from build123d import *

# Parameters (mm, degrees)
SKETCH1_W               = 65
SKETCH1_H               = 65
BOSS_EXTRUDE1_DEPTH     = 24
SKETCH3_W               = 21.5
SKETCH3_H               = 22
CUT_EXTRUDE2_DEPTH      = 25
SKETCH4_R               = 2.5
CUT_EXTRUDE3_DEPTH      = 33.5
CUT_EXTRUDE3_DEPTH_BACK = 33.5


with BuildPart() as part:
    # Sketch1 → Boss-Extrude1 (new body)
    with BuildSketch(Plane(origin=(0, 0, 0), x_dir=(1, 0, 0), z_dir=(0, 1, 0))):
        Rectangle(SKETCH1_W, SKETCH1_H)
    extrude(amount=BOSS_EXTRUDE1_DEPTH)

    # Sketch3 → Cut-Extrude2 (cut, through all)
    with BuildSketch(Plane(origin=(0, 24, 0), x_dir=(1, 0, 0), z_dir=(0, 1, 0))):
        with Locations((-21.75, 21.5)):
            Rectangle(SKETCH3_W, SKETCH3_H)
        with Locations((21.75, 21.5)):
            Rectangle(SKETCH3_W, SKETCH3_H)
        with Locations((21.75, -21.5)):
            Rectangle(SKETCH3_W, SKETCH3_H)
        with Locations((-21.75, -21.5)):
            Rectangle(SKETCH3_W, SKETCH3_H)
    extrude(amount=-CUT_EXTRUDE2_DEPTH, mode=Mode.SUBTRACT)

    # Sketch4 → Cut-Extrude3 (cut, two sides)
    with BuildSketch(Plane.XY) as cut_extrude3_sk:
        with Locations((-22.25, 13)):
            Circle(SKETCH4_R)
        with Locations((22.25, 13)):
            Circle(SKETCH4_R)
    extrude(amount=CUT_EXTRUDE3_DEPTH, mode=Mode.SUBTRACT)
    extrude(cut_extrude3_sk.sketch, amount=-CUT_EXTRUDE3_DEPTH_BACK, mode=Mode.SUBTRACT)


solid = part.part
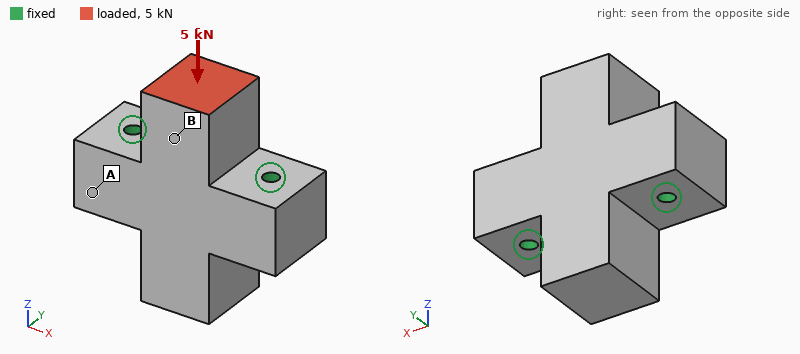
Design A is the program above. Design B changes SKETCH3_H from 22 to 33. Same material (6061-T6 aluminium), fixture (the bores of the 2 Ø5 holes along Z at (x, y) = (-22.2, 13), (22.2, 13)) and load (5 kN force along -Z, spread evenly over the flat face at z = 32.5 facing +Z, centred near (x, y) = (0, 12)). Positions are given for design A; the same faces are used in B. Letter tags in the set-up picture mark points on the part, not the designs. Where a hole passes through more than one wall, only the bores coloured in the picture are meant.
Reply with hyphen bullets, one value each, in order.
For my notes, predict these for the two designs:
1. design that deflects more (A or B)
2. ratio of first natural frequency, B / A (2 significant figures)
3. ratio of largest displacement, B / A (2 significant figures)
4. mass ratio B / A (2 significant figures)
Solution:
- B
- 0.49
- 2.2
- 0.80
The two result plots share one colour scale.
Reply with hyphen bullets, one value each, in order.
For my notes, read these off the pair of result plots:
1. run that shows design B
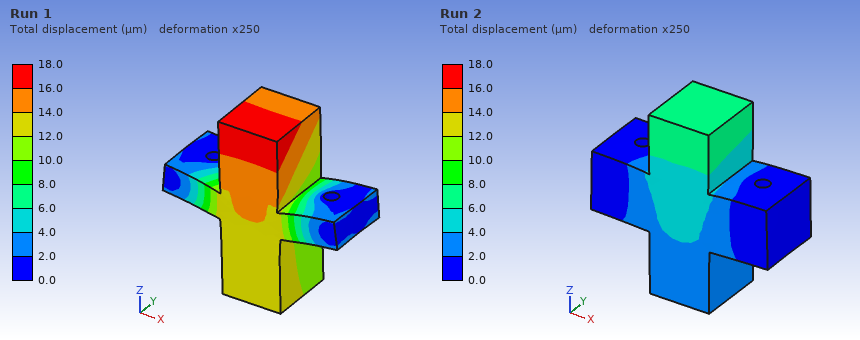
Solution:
- Run 1
